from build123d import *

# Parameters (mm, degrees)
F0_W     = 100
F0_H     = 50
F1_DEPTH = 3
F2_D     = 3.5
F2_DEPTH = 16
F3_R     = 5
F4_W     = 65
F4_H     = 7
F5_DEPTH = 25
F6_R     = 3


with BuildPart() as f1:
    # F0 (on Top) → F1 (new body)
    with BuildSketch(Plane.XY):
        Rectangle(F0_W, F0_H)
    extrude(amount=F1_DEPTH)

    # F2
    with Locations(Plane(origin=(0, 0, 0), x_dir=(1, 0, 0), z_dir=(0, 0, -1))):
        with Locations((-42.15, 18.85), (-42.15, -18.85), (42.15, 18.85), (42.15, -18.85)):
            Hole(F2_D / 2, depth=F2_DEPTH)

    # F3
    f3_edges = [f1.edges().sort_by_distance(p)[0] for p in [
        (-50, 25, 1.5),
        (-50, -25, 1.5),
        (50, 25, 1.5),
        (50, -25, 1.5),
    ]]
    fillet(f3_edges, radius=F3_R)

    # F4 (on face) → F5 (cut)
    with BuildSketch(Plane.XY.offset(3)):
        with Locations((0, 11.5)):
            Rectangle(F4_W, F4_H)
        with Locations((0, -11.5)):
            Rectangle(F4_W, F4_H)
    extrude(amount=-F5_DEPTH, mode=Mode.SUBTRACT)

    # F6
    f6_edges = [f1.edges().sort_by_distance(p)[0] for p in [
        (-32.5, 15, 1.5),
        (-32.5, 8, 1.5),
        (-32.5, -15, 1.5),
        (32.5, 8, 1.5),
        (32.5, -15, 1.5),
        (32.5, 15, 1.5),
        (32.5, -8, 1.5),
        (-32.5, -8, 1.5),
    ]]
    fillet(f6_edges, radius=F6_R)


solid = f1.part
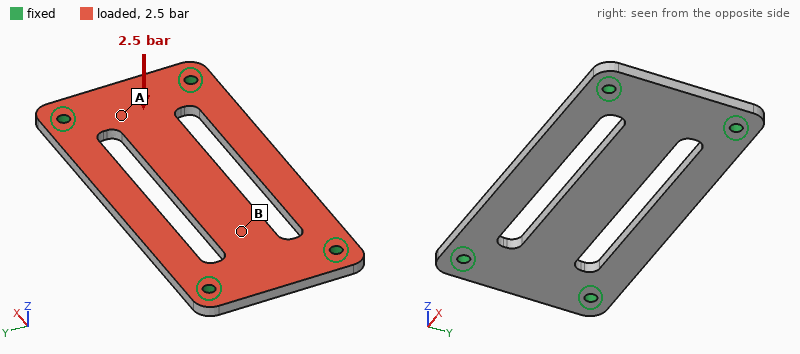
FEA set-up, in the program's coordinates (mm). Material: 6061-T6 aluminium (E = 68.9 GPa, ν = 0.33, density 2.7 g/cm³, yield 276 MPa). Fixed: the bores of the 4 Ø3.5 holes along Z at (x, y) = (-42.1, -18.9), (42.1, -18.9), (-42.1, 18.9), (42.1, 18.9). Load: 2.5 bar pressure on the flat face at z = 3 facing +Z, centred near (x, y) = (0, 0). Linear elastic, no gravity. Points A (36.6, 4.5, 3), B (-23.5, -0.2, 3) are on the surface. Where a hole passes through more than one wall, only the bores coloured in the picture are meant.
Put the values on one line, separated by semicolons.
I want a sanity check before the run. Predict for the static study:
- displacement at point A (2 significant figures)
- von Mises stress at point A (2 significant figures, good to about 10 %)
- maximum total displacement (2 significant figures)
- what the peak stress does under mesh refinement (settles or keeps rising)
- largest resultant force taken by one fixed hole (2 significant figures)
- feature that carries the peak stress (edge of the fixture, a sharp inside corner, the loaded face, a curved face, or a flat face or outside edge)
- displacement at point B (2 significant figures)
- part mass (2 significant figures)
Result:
0.040 mm; 38 MPa; 0.25 mm; keeps rising; 250 N; edge of the fixture; 0.13 mm; 33 g
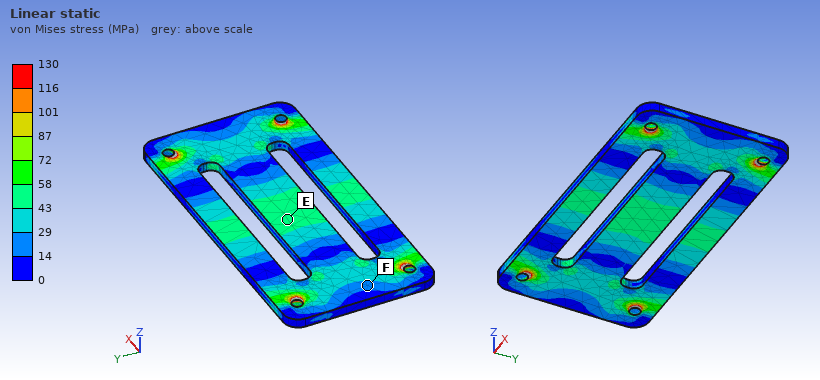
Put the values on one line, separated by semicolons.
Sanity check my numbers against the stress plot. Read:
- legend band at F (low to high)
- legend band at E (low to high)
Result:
14 to 29 MPa; 43 to 58 MPa
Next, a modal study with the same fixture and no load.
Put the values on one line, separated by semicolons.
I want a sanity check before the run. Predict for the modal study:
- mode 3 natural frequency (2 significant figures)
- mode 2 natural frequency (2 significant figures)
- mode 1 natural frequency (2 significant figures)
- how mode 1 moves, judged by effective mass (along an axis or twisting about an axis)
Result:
2600 Hz; 2500 Hz; 2100 Hz; along Z
